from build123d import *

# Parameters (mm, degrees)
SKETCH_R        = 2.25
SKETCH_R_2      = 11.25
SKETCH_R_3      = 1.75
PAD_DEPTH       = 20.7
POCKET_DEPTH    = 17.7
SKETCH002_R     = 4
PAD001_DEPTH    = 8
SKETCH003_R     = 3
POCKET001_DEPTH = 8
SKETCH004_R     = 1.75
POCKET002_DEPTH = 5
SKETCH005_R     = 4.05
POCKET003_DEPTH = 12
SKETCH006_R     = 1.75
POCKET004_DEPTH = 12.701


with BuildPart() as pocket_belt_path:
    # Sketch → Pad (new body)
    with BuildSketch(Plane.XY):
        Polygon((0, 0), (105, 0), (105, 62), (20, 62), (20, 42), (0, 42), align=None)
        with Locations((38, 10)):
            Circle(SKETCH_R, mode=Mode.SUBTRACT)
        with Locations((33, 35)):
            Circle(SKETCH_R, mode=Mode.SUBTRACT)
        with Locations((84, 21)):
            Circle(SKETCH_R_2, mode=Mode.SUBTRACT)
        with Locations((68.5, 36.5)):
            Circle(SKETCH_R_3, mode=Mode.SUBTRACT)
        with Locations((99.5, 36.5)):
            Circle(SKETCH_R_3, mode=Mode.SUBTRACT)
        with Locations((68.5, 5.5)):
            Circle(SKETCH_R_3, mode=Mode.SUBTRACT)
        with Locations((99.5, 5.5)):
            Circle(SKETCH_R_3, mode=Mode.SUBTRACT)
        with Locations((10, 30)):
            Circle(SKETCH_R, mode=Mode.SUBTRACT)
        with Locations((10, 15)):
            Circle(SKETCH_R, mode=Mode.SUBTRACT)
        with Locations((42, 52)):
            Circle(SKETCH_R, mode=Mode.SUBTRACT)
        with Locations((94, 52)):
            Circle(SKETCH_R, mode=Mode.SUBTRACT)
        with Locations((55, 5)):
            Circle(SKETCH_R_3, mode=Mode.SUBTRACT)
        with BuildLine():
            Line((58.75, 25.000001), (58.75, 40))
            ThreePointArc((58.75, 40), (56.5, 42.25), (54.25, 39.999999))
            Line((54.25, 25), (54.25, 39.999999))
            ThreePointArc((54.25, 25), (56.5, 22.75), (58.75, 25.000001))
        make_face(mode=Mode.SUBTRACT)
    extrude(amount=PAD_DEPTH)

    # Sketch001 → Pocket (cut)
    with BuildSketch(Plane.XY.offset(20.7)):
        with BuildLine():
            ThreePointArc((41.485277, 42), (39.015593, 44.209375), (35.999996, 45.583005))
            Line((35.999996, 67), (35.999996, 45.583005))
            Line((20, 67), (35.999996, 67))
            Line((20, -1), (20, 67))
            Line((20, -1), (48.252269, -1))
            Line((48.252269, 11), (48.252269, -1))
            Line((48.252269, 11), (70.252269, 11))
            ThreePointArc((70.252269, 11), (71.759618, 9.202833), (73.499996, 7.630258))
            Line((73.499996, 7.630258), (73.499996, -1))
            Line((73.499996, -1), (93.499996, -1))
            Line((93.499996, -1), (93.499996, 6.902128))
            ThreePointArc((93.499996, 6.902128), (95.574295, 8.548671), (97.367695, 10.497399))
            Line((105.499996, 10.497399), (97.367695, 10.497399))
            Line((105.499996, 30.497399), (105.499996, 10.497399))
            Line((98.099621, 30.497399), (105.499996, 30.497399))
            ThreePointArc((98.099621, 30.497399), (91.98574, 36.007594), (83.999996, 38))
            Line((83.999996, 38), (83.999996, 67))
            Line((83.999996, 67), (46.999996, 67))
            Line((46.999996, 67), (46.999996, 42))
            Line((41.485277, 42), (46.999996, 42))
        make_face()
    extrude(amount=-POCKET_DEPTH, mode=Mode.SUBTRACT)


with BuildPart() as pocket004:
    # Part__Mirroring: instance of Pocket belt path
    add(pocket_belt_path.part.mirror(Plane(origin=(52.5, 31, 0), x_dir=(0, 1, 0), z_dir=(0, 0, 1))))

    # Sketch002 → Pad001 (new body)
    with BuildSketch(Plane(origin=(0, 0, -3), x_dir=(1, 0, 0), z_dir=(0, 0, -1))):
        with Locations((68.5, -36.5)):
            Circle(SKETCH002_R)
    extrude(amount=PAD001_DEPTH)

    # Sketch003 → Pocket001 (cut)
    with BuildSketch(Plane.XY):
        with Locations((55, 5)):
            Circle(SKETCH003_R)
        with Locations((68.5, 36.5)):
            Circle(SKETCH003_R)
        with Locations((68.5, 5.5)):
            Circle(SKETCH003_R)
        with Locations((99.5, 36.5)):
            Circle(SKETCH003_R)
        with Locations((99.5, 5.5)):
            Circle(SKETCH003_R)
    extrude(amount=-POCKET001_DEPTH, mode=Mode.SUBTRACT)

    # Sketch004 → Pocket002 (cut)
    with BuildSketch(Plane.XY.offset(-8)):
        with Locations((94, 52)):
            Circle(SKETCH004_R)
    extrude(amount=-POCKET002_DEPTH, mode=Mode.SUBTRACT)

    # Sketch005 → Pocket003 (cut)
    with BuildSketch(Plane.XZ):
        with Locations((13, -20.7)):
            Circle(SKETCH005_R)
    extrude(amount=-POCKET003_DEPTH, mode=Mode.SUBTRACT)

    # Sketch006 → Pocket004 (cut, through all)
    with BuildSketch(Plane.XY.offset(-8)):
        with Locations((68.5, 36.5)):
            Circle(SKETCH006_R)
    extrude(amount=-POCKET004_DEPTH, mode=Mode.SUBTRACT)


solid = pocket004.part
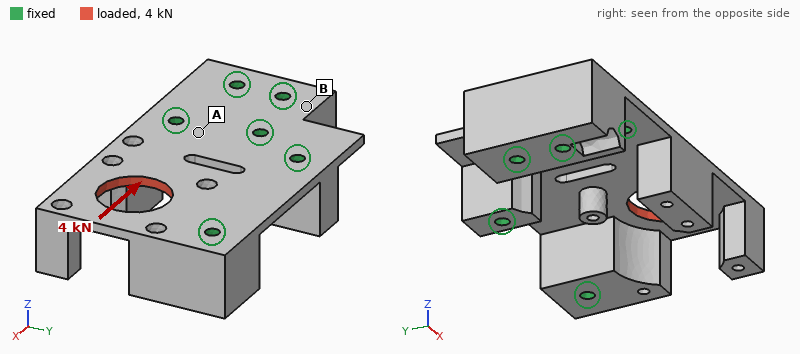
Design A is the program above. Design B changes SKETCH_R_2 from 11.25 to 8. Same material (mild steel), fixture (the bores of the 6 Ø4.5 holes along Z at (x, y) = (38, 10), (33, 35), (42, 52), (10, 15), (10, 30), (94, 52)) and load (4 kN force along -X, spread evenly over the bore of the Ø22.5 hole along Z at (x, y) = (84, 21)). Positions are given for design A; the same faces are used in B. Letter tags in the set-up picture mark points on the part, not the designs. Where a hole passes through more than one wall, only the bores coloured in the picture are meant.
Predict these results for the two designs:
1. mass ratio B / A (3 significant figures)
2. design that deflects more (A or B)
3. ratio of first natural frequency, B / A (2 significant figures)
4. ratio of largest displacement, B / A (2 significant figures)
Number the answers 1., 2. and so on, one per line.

1. 1.01
2. A
3. 1.1
4. 0.82
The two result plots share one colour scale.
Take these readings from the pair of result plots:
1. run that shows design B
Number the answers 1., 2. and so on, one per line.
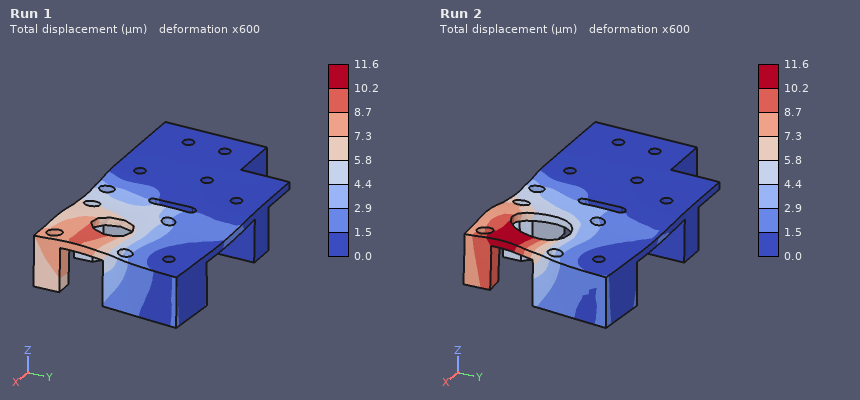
1. Run 1
